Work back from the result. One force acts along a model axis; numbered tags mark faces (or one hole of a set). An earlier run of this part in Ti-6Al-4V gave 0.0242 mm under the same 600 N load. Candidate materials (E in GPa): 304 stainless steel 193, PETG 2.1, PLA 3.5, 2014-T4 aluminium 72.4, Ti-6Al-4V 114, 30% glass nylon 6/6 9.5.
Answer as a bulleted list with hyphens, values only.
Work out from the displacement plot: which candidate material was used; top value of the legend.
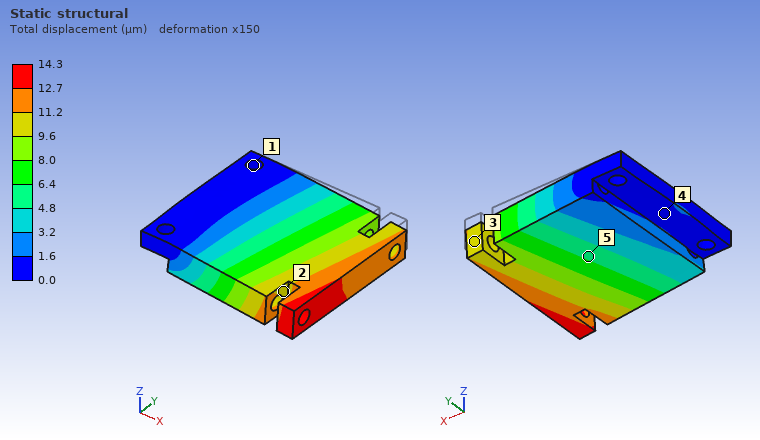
- 304 stainless steel
- 14.3 µm
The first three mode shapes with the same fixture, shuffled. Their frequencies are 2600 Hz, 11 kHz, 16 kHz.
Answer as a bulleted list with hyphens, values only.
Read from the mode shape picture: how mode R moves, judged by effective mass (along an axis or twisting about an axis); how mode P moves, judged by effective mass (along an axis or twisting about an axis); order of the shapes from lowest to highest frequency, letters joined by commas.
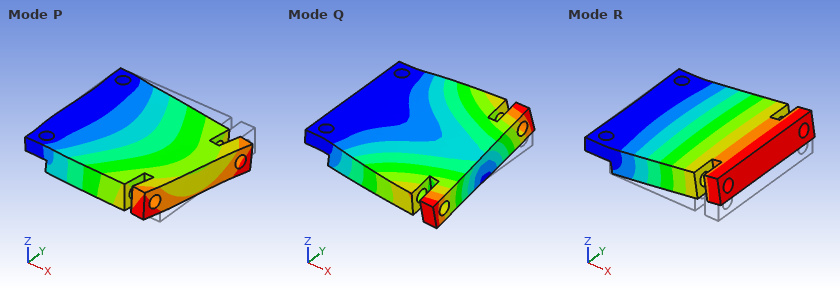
- along Z
- along Y
- R, Q, P
